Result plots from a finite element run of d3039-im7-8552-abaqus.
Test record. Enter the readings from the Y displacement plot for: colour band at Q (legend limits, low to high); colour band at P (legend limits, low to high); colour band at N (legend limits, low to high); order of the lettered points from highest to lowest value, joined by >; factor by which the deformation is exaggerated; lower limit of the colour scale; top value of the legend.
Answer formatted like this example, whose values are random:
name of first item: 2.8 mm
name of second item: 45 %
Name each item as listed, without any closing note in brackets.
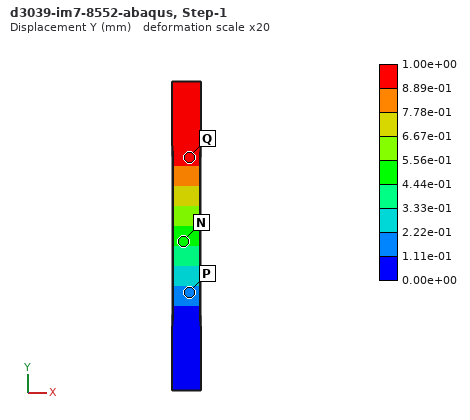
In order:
colour band at Q: 8.89e-01 to 1.00e+00 mm
colour band at P: 1.11e-01 to 2.22e-01 mm
colour band at N: 4.44e-01 to 5.56e-01 mm
order of the lettered points from highest to lowest value, joined by >: Q > N > P
factor by which the deformation is exaggerated: 20
lower limit of the colour scale: 0.00e+00 mm
top value of the legend: 1.00e+00 mm
